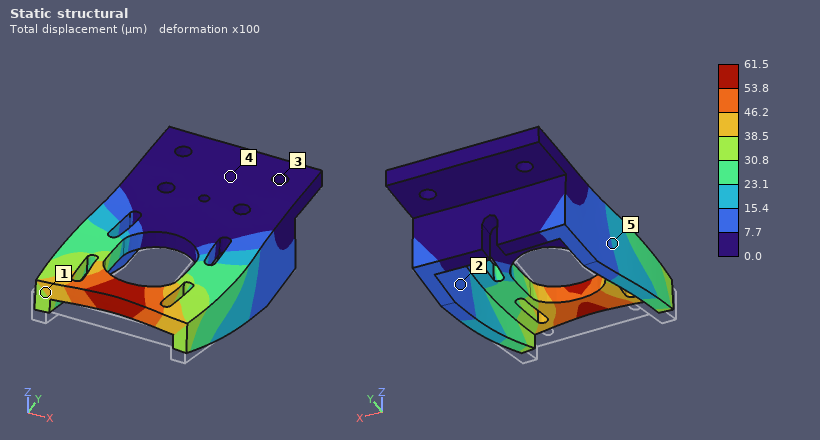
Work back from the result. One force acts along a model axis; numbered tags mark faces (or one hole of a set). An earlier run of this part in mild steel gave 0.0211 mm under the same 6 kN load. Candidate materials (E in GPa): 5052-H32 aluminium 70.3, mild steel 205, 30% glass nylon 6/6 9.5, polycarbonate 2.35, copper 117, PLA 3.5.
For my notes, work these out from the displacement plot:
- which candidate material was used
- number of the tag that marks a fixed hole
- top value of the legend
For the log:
5052-H32 aluminium
3
61.5 µm
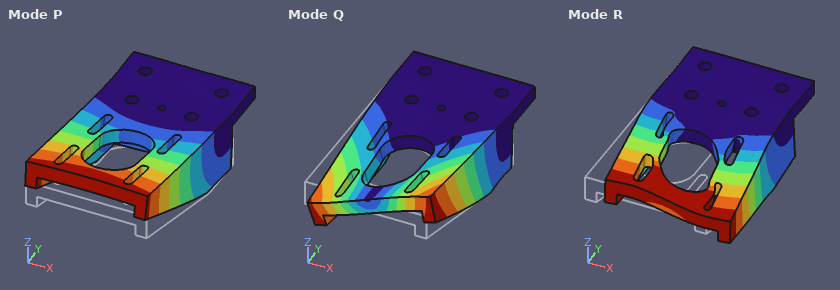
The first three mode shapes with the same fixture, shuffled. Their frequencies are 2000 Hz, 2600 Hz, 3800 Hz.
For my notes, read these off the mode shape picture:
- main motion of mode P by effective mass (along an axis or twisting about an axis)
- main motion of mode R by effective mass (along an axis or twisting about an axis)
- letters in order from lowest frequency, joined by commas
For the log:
along Z
along X
P, Q, R
